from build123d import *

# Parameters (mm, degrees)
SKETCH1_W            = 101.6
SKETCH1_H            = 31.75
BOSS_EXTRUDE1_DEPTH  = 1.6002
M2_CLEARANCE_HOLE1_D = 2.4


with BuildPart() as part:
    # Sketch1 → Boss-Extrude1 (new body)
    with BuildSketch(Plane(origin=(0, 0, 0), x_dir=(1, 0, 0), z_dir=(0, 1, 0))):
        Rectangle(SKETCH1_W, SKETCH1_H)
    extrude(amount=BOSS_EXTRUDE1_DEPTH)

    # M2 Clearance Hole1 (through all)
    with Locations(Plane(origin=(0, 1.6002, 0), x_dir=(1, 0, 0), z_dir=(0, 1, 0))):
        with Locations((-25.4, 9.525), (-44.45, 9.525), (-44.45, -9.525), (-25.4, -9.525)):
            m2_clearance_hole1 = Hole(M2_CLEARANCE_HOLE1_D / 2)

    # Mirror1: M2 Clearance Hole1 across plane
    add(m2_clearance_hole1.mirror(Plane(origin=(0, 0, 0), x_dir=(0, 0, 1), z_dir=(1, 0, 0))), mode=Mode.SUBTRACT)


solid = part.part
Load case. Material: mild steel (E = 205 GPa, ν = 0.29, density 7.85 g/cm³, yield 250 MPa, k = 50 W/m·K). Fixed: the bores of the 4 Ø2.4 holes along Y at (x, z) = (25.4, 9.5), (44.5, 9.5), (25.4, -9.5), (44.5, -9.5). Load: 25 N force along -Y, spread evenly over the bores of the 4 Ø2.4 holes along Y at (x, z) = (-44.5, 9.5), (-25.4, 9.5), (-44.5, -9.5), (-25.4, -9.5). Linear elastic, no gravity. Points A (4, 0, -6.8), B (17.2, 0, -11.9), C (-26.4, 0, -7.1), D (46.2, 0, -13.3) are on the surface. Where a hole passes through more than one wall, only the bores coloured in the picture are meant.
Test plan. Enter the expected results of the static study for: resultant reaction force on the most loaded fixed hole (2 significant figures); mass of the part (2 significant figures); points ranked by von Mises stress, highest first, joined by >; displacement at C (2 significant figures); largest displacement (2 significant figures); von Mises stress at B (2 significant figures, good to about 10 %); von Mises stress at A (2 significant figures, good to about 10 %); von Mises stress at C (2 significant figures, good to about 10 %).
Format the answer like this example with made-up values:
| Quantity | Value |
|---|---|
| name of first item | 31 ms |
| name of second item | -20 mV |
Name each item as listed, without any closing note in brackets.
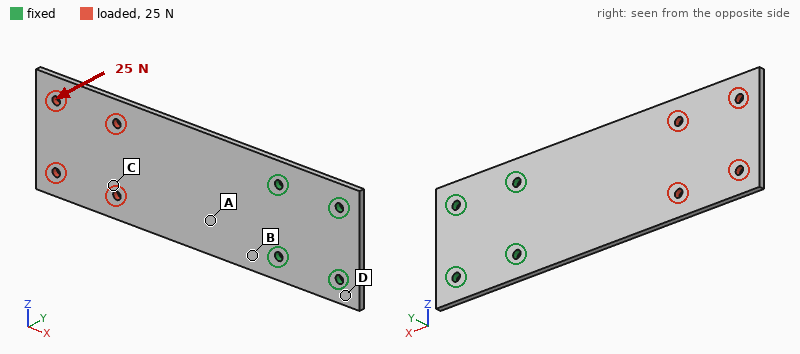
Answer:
| Quantity | Value |
|---|---|
| resultant reaction force on the most loaded fixed hole | 21 N |
| mass of the part | 40 g |
| points ranked by von Mises stress, highest first, joined by > | B > A > C > D |
| displacement at C | 0.64 mm |
| largest displacement | 1.1 mm |
| von Mises stress at B | 94 MPa |
| von Mises stress at A | 69 MPa |
| von Mises stress at C | 20 MPa |
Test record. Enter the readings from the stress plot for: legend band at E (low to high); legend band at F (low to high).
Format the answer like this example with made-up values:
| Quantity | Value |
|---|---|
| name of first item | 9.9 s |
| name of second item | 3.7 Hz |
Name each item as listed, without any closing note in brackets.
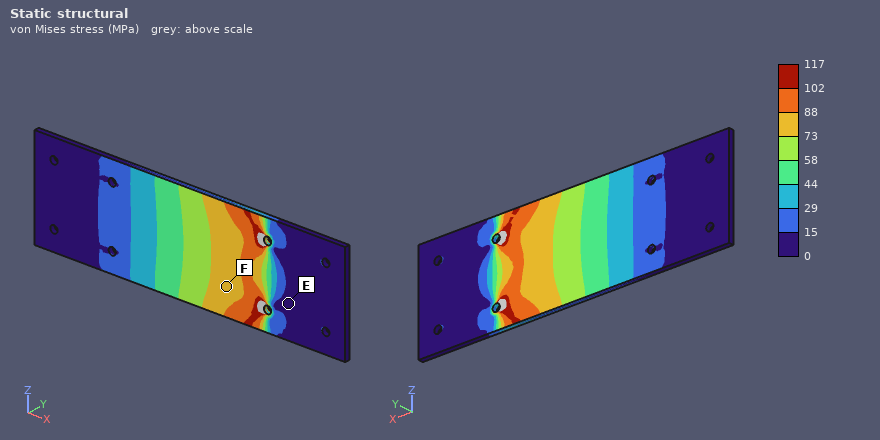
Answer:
| Quantity | Value |
|---|---|
| legend band at E | 0 to 15 MPa |
| legend band at F | 73 to 88 MPa |
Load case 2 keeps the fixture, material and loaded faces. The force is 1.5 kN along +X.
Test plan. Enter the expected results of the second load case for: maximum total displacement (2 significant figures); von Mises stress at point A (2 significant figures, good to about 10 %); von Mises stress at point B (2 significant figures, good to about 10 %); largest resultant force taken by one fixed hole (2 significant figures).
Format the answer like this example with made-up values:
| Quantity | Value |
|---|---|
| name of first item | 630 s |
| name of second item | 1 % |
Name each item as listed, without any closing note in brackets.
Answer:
| Quantity | Value |
|---|---|
| maximum total displacement | 9.9 µm |
| von Mises stress at point A | 30 MPa |
| von Mises stress at point B | 32 MPa |
| largest resultant force taken by one fixed hole | 630 N |
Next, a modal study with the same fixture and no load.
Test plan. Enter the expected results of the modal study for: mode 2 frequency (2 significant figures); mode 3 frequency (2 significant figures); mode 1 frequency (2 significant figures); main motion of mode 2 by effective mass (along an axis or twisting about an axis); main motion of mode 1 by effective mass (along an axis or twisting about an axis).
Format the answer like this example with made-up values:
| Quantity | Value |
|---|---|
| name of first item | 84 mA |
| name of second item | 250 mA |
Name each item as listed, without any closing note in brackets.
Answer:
| Quantity | Value |
|---|---|
| mode 2 frequency | 1200 Hz |
| mode 3 frequency | 1400 Hz |
| mode 1 frequency | 230 Hz |
| main motion of mode 2 by effective mass | twisting about X |
| main motion of mode 1 by effective mass | along Y |
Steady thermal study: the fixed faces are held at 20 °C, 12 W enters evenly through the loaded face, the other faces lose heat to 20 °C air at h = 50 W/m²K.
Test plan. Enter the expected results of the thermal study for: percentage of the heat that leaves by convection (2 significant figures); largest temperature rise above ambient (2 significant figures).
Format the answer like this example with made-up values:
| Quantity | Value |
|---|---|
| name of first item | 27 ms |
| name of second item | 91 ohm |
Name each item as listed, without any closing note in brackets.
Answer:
| Quantity | Value |
|---|---|
| percentage of the heat that leaves by convection | 86 % |
| largest temperature rise above ambient | 85 K |
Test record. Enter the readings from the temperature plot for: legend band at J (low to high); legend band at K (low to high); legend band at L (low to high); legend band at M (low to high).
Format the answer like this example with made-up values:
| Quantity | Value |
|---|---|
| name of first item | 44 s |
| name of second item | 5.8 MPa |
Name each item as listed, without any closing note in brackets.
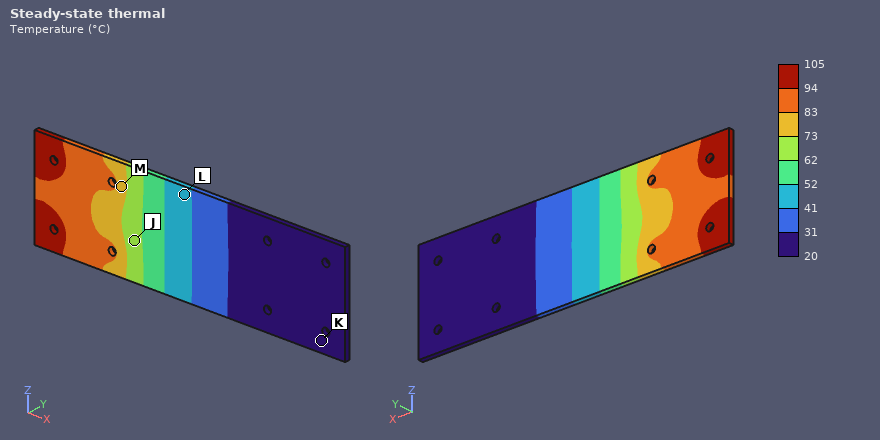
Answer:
| Quantity | Value |
|---|---|
| legend band at J | 62 to 73 °C |
| legend band at K | 20 to 31 °C |
| legend band at L | 41 to 52 °C |
| legend band at M | 73 to 83 °C |
